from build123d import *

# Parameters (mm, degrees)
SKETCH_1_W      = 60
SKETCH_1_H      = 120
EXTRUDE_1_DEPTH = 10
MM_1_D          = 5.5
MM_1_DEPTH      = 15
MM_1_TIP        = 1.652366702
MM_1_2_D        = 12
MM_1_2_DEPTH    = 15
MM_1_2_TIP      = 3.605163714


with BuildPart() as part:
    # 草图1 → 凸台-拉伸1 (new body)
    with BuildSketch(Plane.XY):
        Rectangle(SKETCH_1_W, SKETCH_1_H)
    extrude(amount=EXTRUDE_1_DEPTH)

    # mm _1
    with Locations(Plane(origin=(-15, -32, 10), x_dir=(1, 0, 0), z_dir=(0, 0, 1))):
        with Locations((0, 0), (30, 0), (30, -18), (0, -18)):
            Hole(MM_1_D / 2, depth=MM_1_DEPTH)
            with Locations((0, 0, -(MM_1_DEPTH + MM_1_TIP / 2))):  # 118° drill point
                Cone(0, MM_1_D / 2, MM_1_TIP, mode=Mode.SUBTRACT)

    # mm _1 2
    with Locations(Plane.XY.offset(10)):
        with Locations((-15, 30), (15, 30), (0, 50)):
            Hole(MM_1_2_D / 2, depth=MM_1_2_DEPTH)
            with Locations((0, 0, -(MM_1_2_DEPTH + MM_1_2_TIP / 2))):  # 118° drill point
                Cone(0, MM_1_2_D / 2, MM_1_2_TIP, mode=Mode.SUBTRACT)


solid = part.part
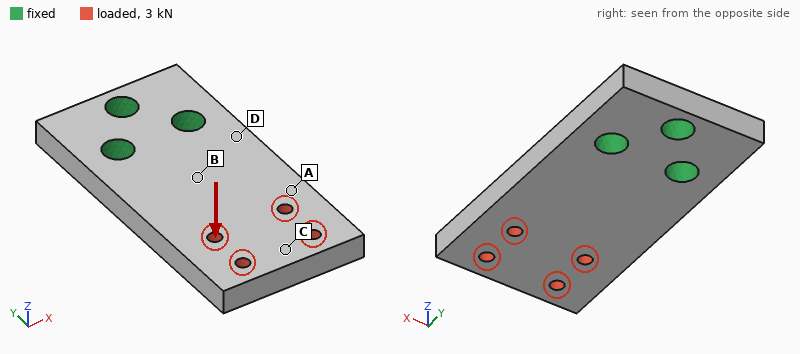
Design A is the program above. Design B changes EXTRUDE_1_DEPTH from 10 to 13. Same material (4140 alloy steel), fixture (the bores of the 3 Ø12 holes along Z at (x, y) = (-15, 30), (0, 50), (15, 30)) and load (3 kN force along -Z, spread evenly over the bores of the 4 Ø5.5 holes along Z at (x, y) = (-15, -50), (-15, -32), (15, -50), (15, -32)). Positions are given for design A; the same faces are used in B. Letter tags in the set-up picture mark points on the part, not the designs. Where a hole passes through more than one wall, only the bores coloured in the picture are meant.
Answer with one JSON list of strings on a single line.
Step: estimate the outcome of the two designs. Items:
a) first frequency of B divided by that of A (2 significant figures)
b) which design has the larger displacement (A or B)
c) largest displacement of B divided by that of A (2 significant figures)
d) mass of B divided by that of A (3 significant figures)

["1.3", "A", "0.47", "1.30"]
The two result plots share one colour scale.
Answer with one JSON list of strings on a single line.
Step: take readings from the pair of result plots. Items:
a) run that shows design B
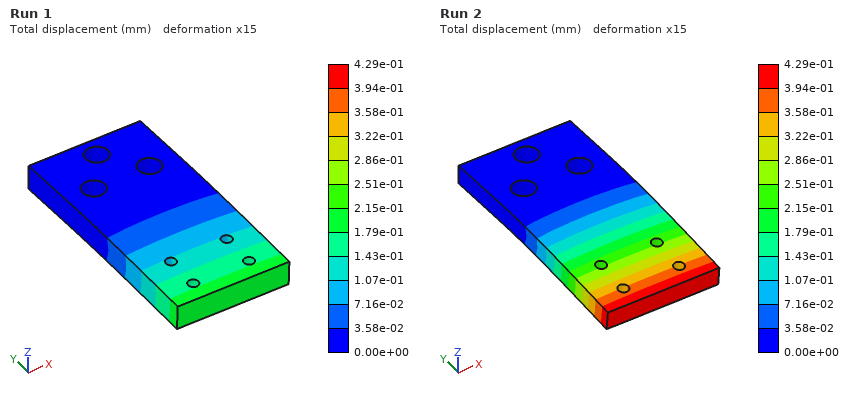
["Run 1"]
